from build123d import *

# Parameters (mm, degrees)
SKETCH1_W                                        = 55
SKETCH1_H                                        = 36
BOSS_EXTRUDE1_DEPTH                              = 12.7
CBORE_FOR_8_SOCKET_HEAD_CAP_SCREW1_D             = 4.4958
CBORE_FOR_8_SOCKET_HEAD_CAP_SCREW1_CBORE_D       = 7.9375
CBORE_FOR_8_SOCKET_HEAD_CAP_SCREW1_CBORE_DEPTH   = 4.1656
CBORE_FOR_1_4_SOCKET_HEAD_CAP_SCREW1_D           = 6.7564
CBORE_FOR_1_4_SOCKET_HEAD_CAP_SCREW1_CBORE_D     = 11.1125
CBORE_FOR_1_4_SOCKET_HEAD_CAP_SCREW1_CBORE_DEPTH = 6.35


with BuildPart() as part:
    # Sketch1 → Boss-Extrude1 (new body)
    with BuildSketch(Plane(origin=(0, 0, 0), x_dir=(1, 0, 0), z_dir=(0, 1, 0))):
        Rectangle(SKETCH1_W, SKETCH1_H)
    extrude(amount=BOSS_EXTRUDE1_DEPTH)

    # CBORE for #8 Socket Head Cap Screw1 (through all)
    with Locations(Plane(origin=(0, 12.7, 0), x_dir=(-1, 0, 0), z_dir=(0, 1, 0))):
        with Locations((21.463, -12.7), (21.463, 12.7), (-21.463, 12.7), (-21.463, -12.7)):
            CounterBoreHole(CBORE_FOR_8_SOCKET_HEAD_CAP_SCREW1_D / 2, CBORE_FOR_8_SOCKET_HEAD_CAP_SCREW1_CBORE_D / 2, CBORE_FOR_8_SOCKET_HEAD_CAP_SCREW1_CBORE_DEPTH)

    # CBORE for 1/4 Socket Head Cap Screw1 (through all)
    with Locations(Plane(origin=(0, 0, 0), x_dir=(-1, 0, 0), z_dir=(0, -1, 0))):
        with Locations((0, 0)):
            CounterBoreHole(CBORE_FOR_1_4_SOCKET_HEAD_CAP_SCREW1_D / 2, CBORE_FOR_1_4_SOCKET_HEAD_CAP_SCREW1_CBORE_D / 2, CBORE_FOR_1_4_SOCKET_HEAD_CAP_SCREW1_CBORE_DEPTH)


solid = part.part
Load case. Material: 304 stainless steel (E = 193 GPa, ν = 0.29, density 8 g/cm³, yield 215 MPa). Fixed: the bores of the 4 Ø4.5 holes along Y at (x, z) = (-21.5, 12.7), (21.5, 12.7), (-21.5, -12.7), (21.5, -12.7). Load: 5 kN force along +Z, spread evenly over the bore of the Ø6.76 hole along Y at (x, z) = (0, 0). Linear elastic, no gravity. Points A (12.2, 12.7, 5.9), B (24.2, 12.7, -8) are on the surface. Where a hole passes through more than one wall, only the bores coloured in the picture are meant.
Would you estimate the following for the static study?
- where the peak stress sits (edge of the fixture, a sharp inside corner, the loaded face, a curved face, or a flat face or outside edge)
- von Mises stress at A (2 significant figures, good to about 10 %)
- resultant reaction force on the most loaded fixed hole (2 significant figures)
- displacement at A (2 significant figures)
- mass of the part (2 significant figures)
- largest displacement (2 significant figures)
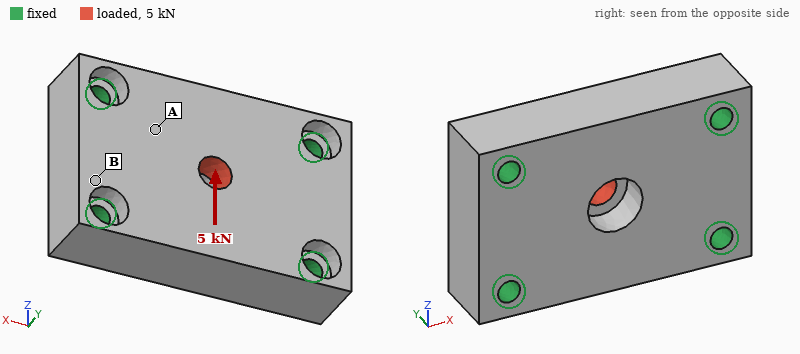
the loaded face
15 MPa
1.6 kN
1.3 µm
180 g
3.4 µm
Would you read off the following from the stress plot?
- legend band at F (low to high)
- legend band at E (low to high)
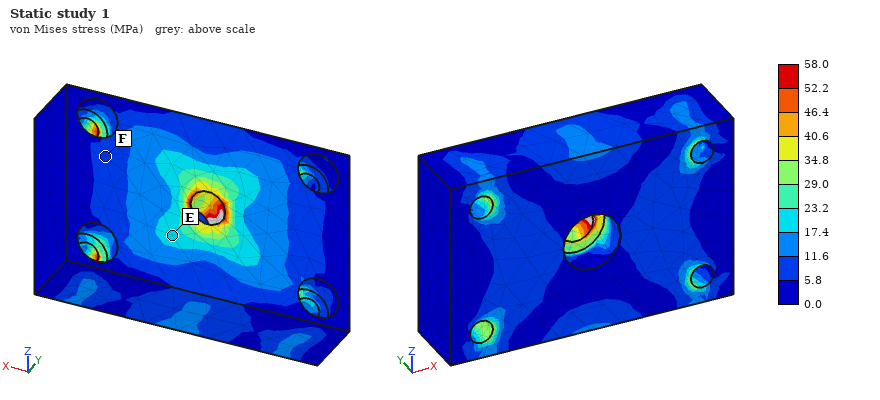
5.8 to 11.6 MPa
17.4 to 23.2 MPa
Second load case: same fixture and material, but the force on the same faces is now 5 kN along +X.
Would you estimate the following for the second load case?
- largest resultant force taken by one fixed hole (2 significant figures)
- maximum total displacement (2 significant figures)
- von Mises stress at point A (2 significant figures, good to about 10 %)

1.3 kN
2.2 µm
12 MPa
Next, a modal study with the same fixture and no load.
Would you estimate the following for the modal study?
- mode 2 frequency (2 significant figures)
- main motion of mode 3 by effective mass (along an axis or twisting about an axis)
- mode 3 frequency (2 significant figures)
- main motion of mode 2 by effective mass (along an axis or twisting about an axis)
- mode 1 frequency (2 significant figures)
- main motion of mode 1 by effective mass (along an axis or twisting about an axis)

26 kHz
along Z
30 kHz
twisting about X
19 kHz
along Y
